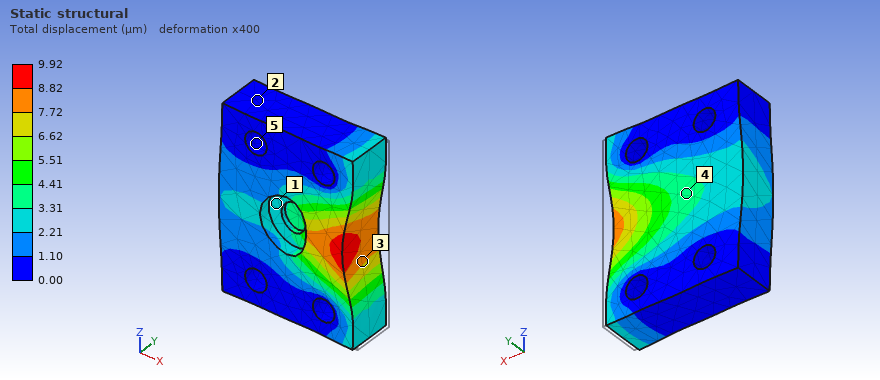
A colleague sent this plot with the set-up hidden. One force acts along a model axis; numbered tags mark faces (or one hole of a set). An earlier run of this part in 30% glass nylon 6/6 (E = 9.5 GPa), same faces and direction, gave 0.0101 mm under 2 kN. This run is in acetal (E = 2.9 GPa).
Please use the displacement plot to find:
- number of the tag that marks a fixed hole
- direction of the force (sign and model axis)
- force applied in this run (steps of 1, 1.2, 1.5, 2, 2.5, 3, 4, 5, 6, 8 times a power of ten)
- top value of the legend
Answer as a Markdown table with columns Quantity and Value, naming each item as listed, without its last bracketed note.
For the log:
| Quantity | Value |
|---|---|
| number of the tag that marks a fixed hole | 5 |
| direction of the force | -X |
| force applied in this run | 600 N |
| top value of the legend | 9.92 µm |
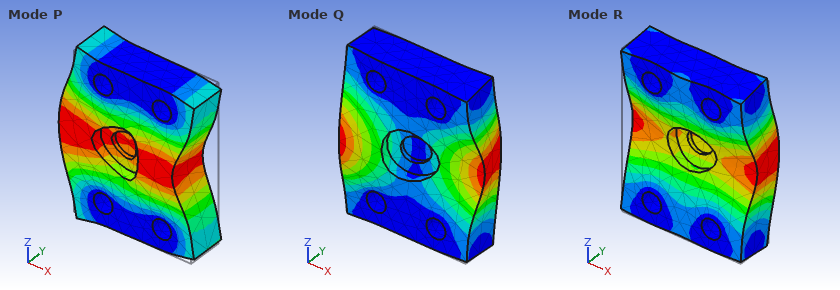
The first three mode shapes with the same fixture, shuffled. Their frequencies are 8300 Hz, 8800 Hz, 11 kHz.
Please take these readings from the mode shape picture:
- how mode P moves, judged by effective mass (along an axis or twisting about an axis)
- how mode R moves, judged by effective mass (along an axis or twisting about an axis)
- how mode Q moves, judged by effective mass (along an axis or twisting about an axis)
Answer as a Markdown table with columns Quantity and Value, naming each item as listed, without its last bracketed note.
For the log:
| Quantity | Value |
|---|---|
| how mode P moves, judged by effective mass | along X |
| how mode R moves, judged by effective mass | along Y |
| how mode Q moves, judged by effective mass | twisting about Z |
